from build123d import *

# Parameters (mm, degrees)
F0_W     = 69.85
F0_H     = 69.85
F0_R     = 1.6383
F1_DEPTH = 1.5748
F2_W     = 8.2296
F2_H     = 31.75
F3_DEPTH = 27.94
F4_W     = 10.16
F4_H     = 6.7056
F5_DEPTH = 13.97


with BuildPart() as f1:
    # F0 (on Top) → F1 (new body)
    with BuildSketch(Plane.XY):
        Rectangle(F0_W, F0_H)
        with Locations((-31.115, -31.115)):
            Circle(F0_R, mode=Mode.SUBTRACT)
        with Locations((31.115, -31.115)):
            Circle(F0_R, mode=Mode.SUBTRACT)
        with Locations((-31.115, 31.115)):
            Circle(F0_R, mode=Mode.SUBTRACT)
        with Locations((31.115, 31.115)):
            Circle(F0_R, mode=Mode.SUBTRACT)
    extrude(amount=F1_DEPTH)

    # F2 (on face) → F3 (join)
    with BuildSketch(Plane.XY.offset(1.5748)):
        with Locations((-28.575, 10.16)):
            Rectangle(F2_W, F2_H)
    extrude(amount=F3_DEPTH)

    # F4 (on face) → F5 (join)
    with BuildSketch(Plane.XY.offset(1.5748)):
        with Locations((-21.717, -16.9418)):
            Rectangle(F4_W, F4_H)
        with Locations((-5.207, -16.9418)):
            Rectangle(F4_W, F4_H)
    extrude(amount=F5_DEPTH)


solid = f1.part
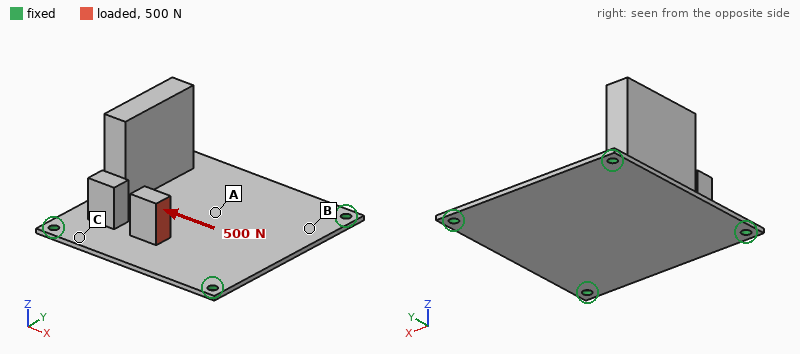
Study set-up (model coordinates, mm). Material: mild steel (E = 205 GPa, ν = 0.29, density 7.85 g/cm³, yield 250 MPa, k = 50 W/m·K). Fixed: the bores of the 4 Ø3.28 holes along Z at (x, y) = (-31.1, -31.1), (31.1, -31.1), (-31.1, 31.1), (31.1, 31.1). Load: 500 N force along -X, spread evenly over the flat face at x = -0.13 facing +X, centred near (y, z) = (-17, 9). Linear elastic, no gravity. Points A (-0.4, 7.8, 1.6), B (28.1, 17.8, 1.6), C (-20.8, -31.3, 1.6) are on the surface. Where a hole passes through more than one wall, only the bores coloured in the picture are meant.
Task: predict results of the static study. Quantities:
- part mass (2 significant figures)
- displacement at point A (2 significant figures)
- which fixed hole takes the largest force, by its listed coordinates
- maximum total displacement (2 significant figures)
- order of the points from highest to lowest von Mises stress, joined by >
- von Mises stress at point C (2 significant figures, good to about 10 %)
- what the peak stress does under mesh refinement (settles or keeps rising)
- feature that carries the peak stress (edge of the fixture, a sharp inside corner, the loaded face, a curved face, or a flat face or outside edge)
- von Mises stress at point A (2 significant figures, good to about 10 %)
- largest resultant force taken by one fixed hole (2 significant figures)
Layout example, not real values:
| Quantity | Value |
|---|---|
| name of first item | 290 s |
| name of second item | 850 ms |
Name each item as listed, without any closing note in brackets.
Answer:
| Quantity | Value |
|---|---|
| part mass | 130 g |
| displacement at point A | 19 µm |
| which fixed hole takes the largest force, by its listed coordinates | (-31.1, -31.1) |
| maximum total displacement | 99 µm |
| order of the points from highest to lowest von Mises stress, joined by > | C > A > B |
| von Mises stress at point C | 36 MPa |
| what the peak stress does under mesh refinement | keeps rising |
| feature that carries the peak stress | edge of the fixture |
| von Mises stress at point A | 25 MPa |
| largest resultant force taken by one fixed hole | 220 N |
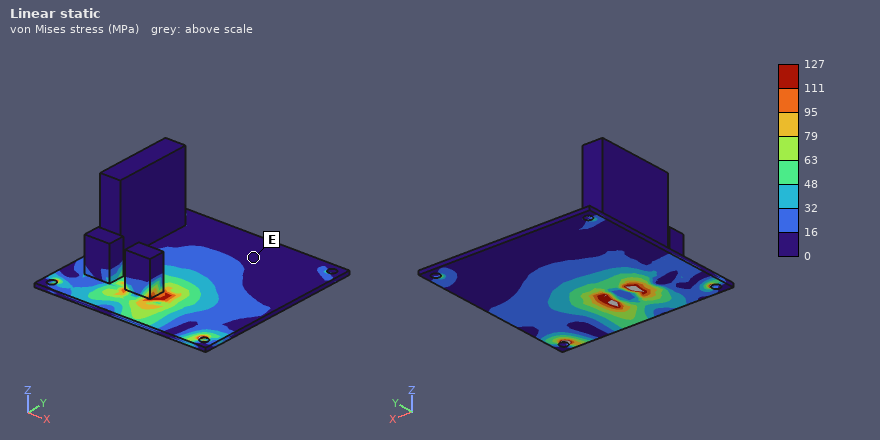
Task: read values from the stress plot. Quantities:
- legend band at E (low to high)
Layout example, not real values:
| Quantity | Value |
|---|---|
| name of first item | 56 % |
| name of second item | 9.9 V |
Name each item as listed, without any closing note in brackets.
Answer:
| Quantity | Value |
|---|---|
| legend band at E | 0 to 16 MPa |
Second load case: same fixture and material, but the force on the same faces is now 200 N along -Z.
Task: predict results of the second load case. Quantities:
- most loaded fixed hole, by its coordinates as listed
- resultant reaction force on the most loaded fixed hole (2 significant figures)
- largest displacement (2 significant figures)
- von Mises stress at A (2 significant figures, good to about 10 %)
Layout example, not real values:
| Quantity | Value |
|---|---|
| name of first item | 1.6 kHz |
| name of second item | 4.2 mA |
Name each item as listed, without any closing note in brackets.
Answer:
| Quantity | Value |
|---|---|
| most loaded fixed hole, by its coordinates as listed | (-31.1, -31.1) |
| resultant reaction force on the most loaded fixed hole | 93 N |
| largest displacement | 0.12 mm |
| von Mises stress at A | 28 MPa |
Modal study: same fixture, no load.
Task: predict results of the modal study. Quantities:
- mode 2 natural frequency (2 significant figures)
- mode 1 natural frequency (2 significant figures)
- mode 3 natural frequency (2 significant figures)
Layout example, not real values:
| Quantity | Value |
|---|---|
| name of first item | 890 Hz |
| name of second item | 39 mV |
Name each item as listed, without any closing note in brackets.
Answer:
| Quantity | Value |
|---|---|
| mode 2 natural frequency | 1100 Hz |
| mode 1 natural frequency | 910 Hz |
| mode 3 natural frequency | 1900 Hz |
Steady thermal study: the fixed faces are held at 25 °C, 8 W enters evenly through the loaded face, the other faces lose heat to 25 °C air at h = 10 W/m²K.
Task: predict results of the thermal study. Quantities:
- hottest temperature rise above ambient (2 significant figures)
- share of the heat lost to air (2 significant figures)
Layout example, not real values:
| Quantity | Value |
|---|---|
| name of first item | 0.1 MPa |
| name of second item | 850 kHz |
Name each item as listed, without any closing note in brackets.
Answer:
| Quantity | Value |
|---|---|
| hottest temperature rise above ambient | 67 K |
| share of the heat lost to air | 27 % |
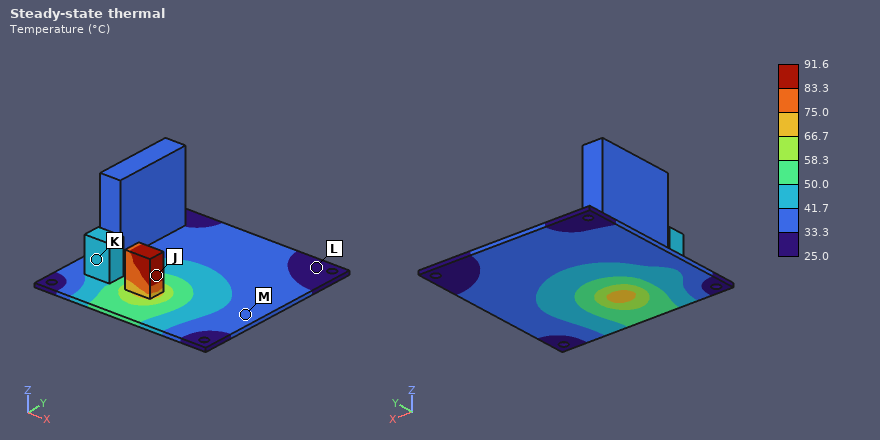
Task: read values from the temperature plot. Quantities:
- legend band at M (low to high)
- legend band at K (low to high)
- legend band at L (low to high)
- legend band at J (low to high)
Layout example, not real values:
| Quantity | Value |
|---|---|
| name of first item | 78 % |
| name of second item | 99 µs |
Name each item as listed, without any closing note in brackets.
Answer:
| Quantity | Value |
|---|---|
| legend band at M | 33.3 to 41.7 °C |
| legend band at K | 41.7 to 50.0 °C |
| legend band at L | 25.0 to 33.3 °C |
| legend band at J | 83.3 to 91.6 °C |
